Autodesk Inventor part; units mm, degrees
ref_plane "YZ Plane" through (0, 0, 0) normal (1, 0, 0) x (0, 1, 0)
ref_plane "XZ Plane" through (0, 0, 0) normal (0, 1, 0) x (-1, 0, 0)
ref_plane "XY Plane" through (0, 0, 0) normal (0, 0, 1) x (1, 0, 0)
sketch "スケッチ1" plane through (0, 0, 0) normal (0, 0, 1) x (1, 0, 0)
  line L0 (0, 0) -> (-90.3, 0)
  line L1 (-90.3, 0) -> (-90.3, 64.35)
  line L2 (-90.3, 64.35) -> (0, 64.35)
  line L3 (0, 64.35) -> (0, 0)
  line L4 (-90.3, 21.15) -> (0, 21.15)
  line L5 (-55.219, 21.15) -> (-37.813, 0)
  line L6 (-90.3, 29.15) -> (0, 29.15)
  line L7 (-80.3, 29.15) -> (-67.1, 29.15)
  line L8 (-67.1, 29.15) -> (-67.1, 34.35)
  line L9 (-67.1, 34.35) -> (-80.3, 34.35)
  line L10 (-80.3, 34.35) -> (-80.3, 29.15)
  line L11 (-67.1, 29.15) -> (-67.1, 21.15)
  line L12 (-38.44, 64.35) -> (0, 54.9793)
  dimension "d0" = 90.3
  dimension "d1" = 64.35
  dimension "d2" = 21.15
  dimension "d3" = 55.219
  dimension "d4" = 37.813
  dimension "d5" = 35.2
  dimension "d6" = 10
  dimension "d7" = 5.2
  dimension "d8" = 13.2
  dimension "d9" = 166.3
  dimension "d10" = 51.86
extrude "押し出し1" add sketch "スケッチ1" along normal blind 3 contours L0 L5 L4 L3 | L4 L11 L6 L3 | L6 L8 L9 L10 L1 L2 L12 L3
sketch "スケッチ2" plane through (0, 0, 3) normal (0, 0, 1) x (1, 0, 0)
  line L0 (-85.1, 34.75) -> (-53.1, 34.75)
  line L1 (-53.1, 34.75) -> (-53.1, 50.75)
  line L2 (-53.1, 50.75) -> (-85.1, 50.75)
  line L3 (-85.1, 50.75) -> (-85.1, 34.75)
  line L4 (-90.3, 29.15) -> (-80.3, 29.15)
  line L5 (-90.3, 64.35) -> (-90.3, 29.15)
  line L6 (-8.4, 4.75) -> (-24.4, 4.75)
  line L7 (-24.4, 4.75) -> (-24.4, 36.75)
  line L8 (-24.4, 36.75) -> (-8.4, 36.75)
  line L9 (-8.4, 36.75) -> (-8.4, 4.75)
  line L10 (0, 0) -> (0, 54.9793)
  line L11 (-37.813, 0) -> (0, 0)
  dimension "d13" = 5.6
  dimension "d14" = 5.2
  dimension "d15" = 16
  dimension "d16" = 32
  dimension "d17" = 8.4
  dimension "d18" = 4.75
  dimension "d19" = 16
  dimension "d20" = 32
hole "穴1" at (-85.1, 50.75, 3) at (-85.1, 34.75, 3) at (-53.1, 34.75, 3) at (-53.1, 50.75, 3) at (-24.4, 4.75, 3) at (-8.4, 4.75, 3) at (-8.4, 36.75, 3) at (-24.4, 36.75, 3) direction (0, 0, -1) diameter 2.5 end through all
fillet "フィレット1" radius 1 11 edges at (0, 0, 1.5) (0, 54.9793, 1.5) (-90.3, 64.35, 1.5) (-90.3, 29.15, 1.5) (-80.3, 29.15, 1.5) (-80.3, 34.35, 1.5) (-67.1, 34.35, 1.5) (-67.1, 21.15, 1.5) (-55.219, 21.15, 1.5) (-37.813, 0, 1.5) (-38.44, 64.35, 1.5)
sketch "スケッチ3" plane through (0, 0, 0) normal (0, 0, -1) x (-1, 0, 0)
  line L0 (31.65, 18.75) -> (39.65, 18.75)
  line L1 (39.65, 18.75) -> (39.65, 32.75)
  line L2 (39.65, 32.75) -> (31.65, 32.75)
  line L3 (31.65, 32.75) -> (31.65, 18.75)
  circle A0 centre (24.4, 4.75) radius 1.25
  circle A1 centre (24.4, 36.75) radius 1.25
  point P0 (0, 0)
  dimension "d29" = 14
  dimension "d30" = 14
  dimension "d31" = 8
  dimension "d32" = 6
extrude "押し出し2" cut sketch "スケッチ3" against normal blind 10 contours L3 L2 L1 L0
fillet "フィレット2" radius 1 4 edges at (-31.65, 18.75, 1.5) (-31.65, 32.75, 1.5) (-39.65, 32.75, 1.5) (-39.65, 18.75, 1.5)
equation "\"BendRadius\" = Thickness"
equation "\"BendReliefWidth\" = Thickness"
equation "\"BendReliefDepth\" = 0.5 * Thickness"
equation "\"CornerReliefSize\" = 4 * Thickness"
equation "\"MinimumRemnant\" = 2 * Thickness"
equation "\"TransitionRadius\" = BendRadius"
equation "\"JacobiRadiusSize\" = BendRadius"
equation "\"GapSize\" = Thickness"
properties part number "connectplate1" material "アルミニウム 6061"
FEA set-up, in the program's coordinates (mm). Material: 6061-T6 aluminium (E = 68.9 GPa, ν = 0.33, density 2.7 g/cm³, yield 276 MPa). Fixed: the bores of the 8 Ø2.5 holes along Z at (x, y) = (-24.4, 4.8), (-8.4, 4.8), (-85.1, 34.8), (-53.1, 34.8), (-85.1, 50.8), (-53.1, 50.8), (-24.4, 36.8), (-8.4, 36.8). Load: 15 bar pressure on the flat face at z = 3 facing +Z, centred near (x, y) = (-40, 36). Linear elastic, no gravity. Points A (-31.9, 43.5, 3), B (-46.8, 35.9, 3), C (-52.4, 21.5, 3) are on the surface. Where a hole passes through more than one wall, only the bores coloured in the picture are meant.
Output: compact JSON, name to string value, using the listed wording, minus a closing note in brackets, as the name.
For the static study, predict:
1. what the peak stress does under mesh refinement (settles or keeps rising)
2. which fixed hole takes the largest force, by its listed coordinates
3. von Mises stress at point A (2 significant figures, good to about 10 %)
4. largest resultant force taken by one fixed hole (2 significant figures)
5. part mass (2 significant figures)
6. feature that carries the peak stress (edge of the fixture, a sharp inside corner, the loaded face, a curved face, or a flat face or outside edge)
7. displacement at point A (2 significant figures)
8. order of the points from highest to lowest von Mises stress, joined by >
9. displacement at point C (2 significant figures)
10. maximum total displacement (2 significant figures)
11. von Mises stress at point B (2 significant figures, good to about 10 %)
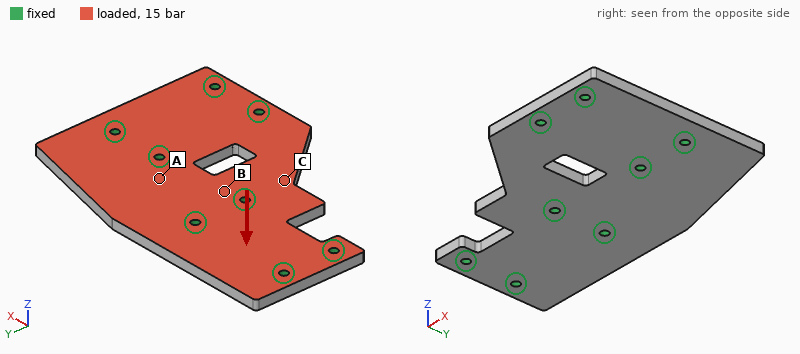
{"what the peak stress does under mesh refinement": "keeps rising", "which fixed hole takes the largest force, by its listed coordinates": "(-53.1, 50.8)", "von Mises stress at point A": "86 MPa", "largest resultant force taken by one fixed hole": "1.3 kN", "part mass": "35 g", "feature that carries the peak stress": "edge of the fixture", "displacement at point A": "0.046 mm", "order of the points from highest to lowest von Mises stress, joined by >": "A > B > C", "displacement at point C": "0.080 mm", "maximum total displacement": "0.25 mm", "von Mises stress at point B": "54 MPa"}
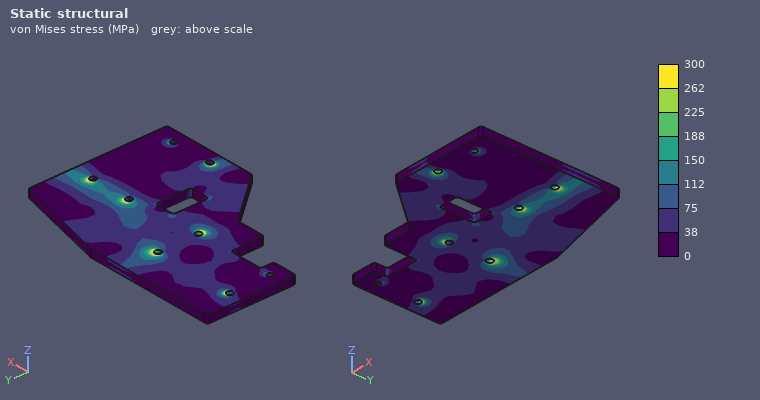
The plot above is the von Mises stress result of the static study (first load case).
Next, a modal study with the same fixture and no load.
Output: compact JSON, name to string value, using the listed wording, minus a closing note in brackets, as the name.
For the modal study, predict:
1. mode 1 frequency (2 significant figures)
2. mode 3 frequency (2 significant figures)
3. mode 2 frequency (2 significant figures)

{"mode 1 frequency": "5500 Hz", "mode 3 frequency": "9200 Hz", "mode 2 frequency": "7800 Hz"}
